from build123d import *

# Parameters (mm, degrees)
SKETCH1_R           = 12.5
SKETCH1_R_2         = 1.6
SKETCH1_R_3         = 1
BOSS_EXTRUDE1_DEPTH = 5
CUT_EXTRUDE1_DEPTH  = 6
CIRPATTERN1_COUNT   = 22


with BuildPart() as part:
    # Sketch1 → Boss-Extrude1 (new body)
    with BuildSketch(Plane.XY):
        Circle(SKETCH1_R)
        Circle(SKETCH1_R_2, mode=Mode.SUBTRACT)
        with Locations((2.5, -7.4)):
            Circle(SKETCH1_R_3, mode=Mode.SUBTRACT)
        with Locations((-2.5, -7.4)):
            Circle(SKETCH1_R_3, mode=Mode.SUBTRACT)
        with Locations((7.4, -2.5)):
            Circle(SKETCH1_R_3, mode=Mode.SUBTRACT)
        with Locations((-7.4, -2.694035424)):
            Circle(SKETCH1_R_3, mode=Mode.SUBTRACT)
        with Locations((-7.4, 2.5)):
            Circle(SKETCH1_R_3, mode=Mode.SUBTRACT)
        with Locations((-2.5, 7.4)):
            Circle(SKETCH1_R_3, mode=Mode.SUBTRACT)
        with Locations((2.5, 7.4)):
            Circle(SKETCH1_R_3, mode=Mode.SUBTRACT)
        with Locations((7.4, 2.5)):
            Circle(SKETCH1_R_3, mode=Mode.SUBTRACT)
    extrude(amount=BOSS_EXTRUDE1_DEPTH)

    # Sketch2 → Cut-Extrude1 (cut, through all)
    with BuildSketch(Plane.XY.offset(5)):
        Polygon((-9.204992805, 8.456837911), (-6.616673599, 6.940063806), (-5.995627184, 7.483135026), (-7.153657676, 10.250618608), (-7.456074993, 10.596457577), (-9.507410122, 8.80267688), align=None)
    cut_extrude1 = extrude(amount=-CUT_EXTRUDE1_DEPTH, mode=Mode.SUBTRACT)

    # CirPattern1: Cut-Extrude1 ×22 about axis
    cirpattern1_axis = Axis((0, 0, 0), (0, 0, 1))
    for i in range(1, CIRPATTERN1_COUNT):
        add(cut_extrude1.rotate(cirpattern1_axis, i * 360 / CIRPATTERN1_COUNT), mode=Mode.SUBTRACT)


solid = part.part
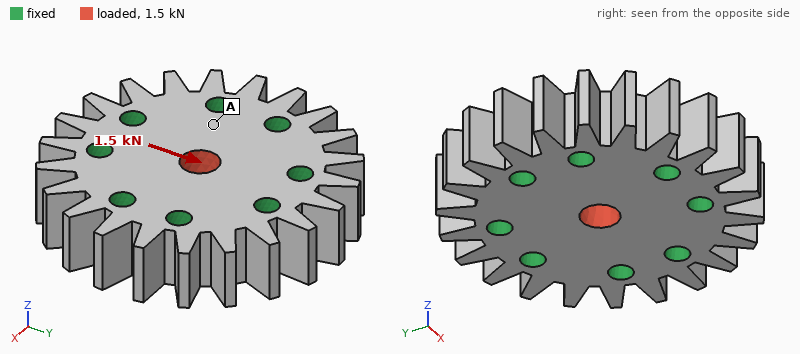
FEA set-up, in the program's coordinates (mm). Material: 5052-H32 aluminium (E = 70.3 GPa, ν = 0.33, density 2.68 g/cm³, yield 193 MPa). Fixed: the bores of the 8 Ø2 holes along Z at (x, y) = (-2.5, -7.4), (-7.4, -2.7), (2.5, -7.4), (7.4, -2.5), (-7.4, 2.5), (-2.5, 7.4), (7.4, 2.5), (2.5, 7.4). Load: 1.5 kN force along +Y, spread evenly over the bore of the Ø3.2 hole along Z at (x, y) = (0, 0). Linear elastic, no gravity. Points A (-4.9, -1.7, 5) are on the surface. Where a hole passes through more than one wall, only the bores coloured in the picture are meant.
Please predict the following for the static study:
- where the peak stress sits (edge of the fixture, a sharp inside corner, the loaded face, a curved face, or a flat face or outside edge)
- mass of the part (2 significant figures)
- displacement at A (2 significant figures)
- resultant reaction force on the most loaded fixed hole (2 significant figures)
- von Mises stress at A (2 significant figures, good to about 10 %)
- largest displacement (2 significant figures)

the loaded face
4.6 g
0.28 µm
310 N
7.3 MPa
1.7 µm
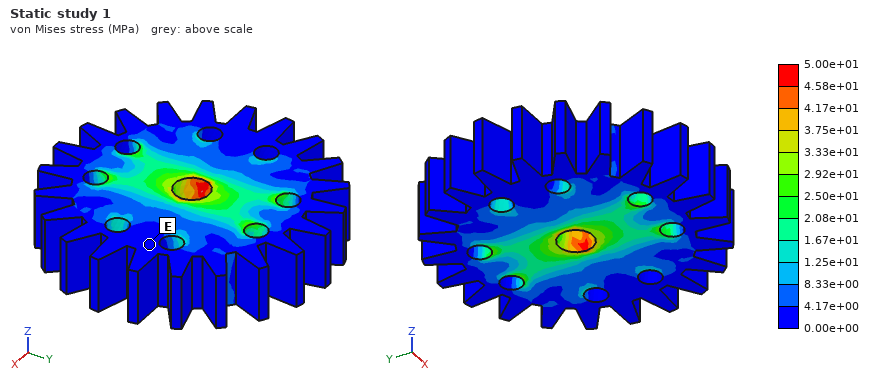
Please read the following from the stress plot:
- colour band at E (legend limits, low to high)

0.00e+00 to 4.17e+00 MPa
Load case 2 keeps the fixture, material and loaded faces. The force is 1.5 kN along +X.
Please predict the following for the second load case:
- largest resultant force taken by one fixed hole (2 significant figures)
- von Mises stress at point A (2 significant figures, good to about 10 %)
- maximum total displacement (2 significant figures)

320 N
18 MPa
1.7 µm
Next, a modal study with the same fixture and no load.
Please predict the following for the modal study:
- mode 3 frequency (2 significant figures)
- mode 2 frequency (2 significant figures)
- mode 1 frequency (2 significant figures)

130 kHz
130 kHz
120 kHz
